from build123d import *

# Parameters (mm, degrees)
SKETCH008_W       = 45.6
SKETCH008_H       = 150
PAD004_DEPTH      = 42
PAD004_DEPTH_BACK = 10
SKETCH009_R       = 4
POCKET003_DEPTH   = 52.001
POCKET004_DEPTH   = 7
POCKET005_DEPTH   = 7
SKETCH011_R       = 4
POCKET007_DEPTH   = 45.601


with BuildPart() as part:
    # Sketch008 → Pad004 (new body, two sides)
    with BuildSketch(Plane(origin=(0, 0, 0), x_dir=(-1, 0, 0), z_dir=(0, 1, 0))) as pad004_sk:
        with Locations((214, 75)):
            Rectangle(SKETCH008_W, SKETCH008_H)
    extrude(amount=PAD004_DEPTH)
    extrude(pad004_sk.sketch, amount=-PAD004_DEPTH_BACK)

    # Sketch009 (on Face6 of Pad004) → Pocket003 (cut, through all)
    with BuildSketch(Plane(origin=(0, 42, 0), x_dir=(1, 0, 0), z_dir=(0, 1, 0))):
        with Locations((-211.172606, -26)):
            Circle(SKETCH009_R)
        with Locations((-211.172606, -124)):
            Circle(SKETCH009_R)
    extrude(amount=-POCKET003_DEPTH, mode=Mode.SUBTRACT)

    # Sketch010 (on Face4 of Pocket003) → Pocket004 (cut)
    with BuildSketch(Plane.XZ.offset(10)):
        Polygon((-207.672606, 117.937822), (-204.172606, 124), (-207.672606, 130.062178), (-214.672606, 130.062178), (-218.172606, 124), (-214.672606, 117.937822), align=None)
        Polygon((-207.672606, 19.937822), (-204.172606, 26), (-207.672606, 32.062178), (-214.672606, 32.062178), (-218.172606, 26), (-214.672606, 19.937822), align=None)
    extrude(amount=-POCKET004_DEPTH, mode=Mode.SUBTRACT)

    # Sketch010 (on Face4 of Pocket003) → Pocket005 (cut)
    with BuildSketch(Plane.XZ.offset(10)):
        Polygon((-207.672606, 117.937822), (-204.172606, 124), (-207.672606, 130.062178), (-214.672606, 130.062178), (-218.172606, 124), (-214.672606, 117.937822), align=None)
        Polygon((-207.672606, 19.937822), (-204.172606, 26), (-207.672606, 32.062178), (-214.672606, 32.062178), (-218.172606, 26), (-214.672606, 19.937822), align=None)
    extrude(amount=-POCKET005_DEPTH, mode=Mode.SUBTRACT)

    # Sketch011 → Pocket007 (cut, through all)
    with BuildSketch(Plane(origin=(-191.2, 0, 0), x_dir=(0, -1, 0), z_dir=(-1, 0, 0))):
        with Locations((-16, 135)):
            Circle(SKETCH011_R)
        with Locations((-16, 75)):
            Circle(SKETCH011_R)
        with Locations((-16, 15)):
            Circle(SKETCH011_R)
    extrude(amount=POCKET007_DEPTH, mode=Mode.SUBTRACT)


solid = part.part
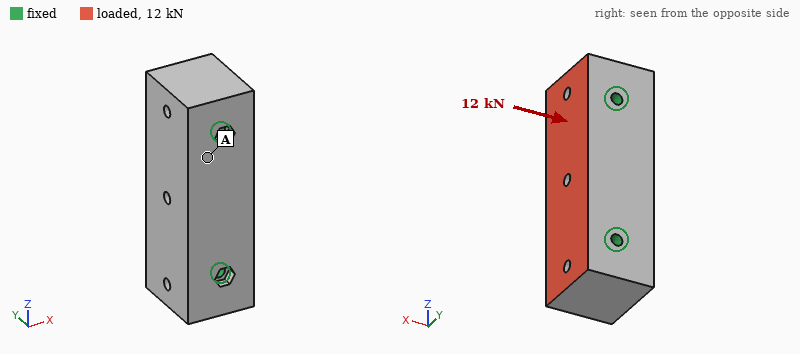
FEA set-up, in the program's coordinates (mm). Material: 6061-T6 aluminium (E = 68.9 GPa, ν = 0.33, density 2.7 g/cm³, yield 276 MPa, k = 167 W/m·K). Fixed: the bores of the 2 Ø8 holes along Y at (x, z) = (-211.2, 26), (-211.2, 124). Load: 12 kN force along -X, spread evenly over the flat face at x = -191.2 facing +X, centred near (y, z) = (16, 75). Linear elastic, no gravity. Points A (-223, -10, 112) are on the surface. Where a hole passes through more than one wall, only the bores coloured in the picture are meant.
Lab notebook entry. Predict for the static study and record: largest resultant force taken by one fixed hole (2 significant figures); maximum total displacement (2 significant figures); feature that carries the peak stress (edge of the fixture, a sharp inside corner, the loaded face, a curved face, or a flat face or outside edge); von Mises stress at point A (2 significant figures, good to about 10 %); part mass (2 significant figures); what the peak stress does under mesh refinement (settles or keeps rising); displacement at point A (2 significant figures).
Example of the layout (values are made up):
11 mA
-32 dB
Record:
6.0 kN
4.5 µm
edge of the fixture
2.4 MPa
920 g
keeps rising
1.9 µm
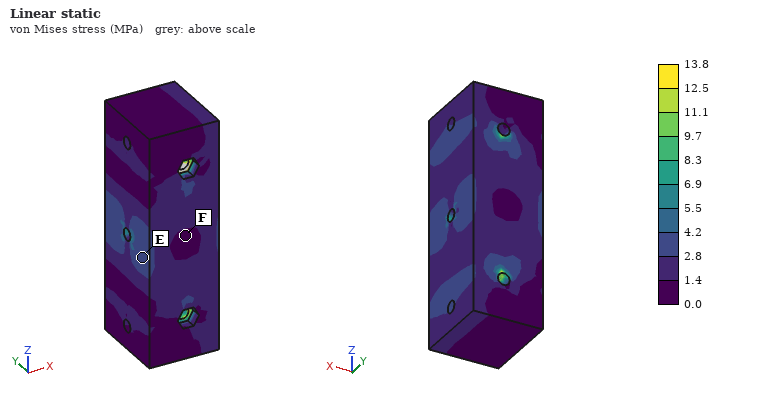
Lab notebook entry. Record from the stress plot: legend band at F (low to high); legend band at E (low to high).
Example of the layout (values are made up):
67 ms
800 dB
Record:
0.0 to 1.4 MPa
2.8 to 4.2 MPa
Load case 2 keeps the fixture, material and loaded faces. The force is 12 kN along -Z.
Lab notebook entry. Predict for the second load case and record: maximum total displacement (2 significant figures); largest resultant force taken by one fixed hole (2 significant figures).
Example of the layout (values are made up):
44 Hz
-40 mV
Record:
4.4 µm
6.4 kN
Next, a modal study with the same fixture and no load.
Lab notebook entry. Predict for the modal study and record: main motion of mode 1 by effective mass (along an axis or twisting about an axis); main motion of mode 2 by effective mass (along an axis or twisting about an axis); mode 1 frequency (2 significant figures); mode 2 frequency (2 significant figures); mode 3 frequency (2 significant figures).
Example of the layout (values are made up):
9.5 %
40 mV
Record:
along X
along Y
8800 Hz
11 kHz
12 kHz
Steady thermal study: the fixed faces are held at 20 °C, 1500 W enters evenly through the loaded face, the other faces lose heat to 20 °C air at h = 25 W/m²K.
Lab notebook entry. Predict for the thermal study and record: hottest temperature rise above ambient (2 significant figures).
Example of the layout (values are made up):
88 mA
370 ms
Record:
59 K
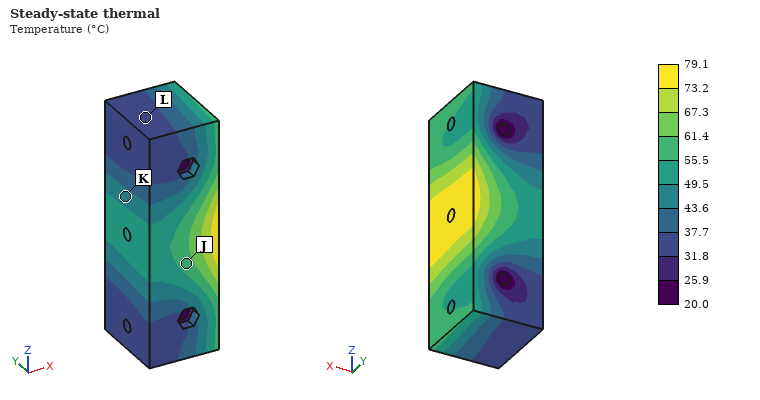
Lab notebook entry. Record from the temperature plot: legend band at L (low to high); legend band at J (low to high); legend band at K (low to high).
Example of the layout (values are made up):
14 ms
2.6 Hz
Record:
31.8 to 37.7 °C
55.5 to 61.4 °C
43.6 to 49.5 °C
